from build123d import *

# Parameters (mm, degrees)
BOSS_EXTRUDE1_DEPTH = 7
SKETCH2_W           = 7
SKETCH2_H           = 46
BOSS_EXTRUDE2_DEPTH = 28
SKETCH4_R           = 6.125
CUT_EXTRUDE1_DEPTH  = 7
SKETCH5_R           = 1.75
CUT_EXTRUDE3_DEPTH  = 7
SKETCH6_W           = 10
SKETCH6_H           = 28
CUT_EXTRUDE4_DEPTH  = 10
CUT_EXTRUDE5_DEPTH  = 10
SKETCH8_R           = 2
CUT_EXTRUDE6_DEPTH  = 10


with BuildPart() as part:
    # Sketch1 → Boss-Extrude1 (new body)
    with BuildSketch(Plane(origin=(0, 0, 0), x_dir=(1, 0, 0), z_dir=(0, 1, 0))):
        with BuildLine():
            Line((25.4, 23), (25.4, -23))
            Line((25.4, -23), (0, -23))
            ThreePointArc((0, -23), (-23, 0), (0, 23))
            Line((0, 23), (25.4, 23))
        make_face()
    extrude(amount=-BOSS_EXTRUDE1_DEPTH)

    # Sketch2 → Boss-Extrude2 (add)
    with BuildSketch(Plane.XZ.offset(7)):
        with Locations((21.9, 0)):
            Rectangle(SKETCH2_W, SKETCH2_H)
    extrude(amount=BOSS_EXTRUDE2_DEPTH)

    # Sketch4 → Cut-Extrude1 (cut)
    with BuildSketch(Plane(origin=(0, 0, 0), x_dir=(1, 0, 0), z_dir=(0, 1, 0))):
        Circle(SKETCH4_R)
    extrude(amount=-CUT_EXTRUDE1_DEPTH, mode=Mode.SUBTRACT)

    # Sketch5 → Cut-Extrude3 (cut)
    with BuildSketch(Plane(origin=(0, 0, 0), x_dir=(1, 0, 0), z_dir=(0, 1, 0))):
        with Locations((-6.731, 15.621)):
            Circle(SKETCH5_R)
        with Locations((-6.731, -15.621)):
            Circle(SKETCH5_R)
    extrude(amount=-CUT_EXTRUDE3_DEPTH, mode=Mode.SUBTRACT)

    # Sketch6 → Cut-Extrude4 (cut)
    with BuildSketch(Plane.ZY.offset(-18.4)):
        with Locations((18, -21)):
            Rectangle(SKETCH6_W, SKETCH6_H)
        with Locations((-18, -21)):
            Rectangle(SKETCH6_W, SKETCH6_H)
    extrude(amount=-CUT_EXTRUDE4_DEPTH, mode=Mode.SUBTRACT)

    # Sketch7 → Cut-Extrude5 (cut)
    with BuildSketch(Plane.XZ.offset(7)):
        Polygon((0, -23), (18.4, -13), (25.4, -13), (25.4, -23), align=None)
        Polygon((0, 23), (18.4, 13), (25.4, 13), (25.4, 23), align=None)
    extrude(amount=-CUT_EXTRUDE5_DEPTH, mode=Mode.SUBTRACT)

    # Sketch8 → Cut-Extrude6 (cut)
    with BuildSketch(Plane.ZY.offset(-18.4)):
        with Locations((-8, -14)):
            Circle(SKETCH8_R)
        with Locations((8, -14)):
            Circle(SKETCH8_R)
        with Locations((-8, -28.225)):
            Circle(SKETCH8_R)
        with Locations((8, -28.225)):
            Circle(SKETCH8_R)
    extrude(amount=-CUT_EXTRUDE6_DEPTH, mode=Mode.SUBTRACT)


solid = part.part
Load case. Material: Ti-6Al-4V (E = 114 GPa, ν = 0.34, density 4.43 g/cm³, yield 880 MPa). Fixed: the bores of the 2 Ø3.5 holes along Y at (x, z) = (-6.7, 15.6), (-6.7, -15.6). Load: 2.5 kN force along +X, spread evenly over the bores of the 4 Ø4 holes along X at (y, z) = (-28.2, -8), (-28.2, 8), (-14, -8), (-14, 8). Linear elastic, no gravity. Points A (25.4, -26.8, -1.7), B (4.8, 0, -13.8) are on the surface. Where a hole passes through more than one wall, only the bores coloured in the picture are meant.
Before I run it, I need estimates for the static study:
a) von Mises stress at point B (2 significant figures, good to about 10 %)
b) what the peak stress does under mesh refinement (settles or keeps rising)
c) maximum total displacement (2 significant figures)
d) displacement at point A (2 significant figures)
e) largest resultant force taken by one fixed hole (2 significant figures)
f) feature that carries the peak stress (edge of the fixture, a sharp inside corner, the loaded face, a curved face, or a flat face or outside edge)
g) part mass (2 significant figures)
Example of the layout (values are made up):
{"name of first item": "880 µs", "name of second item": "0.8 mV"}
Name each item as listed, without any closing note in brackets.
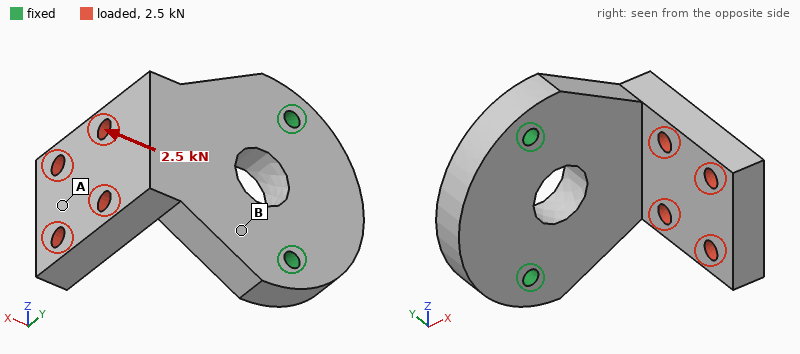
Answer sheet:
{"von Mises stress at point B": "160 MPa", "what the peak stress does under mesh refinement": "keeps rising", "maximum total displacement": "0.59 mm", "displacement at point A": "0.46 mm", "largest resultant force taken by one fixed hole": "1.3 kN", "feature that carries the peak stress": "edge of the fixture", "part mass": "69 g"}
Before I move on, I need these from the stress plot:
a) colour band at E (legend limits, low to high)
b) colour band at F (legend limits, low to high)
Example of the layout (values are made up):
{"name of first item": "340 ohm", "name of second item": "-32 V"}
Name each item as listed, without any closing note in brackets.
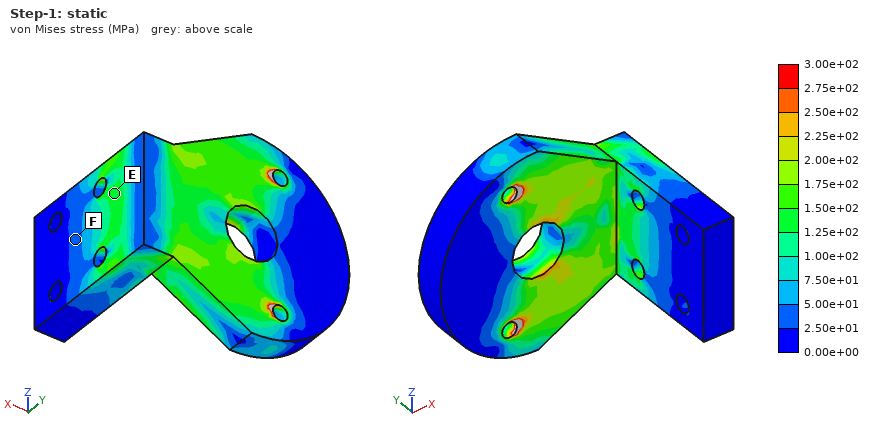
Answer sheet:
{"colour band at E": "1.25e+02 to 1.50e+02 MPa", "colour band at F": "2.50e+01 to 5.00e+01 MPa"}
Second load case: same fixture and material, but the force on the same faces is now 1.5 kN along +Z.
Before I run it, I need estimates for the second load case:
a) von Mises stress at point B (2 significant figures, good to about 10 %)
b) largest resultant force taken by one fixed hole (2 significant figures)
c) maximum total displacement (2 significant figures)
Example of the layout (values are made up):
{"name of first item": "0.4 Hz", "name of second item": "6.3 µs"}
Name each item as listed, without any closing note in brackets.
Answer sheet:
{"von Mises stress at point B": "48 MPa", "largest resultant force taken by one fixed hole": "1.7 kN", "maximum total displacement": "0.13 mm"}
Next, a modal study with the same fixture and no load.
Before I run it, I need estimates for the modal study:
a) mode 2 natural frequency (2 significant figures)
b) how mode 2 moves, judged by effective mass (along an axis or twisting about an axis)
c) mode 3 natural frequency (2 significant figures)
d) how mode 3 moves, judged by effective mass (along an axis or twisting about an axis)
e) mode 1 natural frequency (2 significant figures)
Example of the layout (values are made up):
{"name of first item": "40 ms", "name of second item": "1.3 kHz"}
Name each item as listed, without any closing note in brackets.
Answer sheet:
{"mode 2 natural frequency": "4300 Hz", "how mode 2 moves, judged by effective mass": "along Z", "mode 3 natural frequency": "5800 Hz", "how mode 3 moves, judged by effective mass": "along Y", "mode 1 natural frequency": "2200 Hz"}
